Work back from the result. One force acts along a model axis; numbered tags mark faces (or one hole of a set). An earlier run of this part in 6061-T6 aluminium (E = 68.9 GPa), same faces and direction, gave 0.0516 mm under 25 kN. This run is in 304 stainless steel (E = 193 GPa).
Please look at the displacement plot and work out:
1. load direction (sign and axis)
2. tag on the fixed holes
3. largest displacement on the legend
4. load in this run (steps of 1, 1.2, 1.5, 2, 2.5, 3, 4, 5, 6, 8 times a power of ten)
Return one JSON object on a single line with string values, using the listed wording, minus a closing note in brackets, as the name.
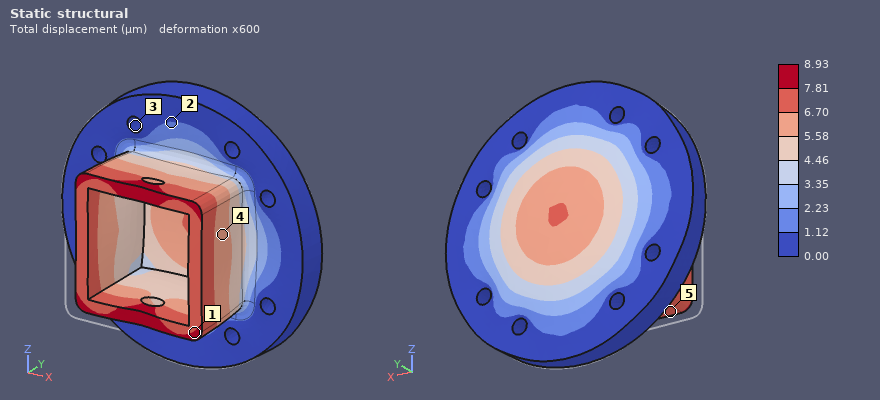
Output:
{"load direction": "+Y", "tag on the fixed holes": "3", "largest displacement on the legend": "8.93 µm", "load in this run": "12 kN"}
